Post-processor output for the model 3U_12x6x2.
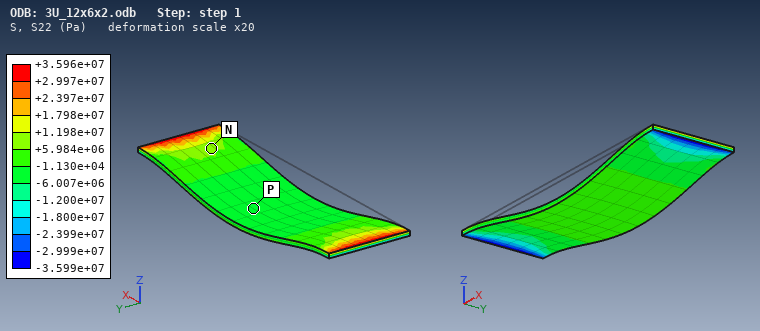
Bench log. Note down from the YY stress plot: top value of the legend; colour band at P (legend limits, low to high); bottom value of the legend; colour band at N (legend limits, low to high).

+3.596e+07 Pa
-6.007e+06 to -1.130e+04 Pa
-3.599e+07 Pa
+5.984e+06 to +1.198e+07 Pa
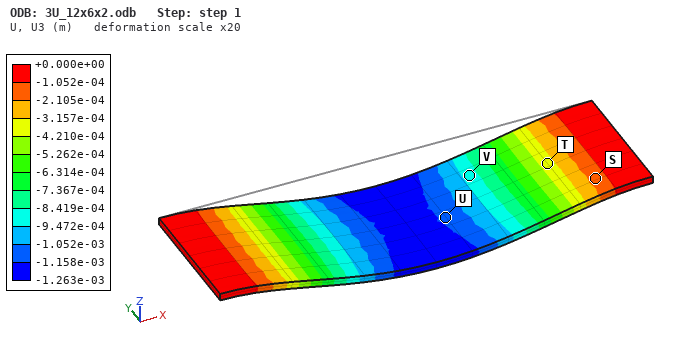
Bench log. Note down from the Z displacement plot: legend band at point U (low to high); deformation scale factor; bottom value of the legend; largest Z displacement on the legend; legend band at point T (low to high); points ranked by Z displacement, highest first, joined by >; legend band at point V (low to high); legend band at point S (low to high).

-1.158e-03 to -1.052e-03 m
20
-1.263e-03 m
+0.000e+00 m
-4.210e-04 to -3.157e-04 m
S > T > V > U
-9.472e-04 to -8.419e-04 m
-2.105e-04 to -1.052e-04 m
